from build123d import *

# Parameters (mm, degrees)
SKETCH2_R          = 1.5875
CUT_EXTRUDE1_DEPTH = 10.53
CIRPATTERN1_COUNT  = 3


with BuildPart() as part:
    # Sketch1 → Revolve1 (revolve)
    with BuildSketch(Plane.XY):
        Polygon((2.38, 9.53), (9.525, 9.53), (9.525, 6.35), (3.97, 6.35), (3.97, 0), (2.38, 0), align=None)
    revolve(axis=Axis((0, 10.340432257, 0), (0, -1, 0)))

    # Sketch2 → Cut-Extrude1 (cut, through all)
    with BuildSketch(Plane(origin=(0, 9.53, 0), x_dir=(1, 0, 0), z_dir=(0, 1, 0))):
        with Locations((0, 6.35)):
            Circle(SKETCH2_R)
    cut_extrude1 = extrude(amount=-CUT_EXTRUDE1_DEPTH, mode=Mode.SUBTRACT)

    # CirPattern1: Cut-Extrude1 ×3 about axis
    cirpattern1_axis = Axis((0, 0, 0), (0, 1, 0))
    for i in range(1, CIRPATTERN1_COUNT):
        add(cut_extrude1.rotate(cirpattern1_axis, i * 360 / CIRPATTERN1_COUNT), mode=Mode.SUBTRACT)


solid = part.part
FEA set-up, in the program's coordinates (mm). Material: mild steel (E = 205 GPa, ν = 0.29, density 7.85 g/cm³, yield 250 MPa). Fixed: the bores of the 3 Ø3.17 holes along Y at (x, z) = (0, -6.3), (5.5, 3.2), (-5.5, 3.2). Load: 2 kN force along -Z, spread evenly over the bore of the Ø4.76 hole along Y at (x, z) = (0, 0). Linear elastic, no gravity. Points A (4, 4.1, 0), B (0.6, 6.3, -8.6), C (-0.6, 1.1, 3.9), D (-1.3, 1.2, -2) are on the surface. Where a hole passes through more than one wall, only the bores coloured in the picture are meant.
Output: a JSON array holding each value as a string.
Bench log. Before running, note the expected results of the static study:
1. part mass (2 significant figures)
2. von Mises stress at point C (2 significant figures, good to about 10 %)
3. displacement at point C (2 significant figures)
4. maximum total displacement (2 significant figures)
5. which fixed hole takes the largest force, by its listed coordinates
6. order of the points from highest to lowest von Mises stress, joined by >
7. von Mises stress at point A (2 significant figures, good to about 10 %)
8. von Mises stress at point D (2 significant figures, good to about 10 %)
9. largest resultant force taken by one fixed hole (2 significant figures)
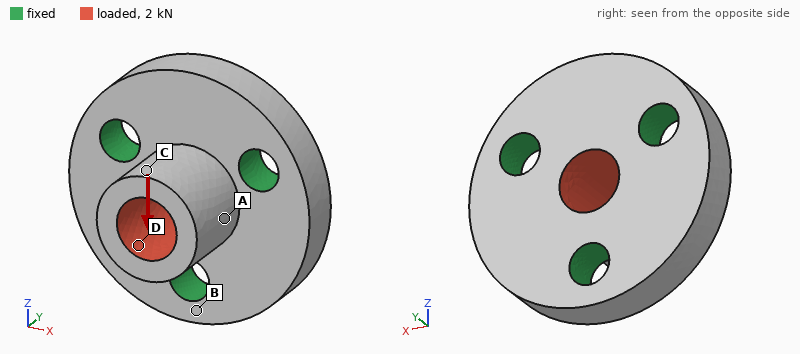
["7.7 g", "31 MPa", "7.1 µm", "8.0 µm", "(0, -6.3)", "A > D > C > B", "63 MPa", "44 MPa", "970 N"]
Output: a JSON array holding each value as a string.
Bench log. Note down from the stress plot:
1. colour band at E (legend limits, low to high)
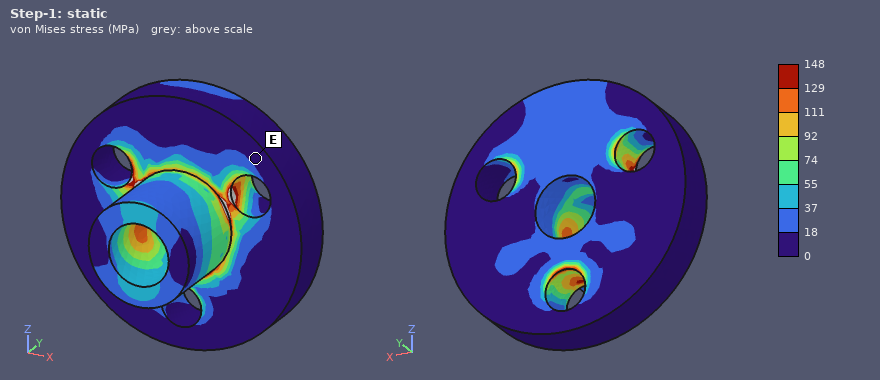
["0 to 18 MPa"]
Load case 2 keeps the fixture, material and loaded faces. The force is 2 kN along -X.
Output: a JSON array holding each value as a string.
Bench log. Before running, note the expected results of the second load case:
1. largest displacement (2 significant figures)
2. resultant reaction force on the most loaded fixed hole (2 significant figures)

["7.8 µm", "890 N"]
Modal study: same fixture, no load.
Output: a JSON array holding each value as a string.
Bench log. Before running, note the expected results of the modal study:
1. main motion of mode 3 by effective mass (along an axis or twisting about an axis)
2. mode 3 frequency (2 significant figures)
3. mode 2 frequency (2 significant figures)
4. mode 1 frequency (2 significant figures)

["along Y", "75 kHz", "59 kHz", "59 kHz"]
